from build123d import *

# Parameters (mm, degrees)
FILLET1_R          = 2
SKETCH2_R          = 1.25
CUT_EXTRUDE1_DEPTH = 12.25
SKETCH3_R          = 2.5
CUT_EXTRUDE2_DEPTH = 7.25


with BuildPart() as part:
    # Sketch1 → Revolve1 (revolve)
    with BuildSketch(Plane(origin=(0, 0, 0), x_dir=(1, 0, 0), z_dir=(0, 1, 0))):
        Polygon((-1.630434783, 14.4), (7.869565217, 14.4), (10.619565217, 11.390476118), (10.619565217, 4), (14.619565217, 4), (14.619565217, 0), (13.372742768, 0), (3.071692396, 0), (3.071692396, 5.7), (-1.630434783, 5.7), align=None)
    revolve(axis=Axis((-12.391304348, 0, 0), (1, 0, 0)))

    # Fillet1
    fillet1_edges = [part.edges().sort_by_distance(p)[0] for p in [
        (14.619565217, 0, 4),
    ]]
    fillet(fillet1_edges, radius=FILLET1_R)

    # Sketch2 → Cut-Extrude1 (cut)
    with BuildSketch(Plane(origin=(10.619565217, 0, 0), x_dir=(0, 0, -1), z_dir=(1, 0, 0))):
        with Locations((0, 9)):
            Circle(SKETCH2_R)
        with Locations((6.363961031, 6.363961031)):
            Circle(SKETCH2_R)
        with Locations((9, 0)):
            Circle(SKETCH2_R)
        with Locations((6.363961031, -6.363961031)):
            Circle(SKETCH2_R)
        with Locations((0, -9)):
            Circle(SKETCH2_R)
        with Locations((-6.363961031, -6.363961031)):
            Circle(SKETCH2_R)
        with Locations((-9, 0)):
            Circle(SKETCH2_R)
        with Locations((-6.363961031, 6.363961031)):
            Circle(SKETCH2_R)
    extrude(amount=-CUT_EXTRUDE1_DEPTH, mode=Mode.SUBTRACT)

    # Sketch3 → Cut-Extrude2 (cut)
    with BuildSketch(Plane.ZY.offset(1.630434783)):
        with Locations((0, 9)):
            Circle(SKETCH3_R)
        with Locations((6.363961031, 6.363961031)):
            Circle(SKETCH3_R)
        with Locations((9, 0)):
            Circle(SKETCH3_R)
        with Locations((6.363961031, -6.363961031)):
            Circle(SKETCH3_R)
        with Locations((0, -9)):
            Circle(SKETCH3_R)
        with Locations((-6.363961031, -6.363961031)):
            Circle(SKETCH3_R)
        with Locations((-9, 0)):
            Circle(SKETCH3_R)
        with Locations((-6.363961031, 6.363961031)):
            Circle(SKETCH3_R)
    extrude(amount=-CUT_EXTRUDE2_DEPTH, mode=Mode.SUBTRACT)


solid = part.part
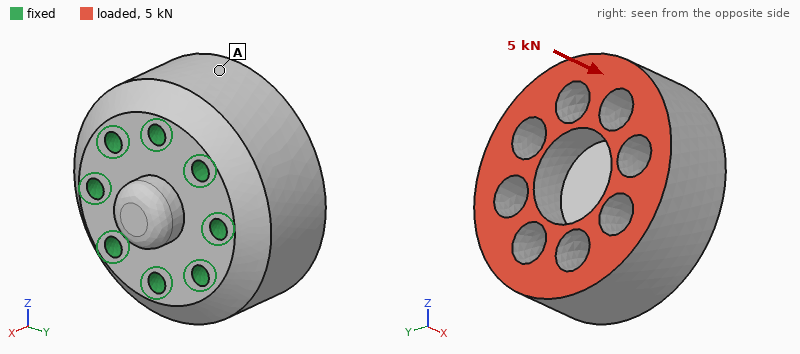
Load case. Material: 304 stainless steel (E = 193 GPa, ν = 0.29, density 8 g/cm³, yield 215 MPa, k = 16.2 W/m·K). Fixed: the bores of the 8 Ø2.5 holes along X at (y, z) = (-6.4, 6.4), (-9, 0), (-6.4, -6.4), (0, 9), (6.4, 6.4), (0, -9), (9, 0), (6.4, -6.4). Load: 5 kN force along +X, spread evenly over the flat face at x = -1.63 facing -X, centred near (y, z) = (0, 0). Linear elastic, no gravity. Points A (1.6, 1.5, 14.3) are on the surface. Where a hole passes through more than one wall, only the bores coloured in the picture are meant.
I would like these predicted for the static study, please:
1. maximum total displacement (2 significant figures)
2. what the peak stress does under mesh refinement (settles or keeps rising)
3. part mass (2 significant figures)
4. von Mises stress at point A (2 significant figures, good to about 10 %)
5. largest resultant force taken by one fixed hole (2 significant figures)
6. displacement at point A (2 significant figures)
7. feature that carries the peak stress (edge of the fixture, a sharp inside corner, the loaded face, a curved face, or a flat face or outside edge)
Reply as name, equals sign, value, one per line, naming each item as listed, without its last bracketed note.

maximum total displacement = 1.4 µm
what the peak stress does under mesh refinement = keeps rising
part mass = 48 g
von Mises stress at point A = 13 MPa
largest resultant force taken by one fixed hole = 630 N
displacement at point A = 1.1 µm
feature that carries the peak stress = edge of the fixture
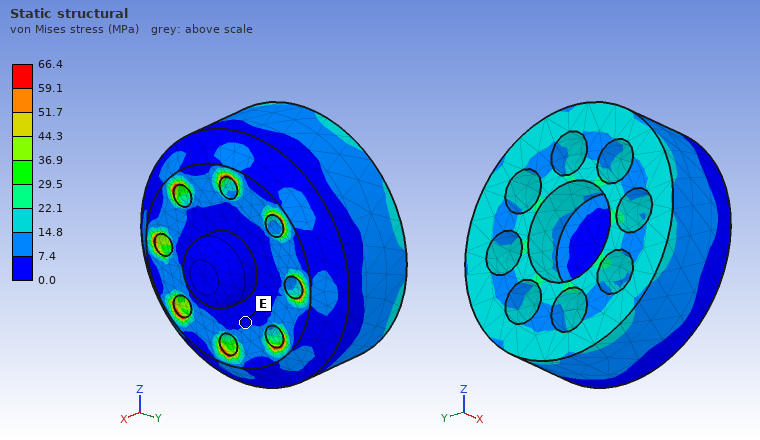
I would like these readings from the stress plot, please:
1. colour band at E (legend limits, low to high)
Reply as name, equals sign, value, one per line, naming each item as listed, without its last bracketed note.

colour band at E = 0.0 to 7.4 MPa
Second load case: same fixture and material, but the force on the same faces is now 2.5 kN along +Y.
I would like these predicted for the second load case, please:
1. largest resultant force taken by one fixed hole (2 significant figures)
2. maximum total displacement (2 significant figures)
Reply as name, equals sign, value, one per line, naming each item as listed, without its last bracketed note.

largest resultant force taken by one fixed hole = 530 N
maximum total displacement = 3.1 µm
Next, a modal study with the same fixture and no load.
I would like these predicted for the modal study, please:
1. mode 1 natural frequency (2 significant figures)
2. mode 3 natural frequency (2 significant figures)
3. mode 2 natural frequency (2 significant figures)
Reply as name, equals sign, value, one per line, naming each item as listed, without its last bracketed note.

mode 1 natural frequency = 47 kHz
mode 3 natural frequency = 51 kHz
mode 2 natural frequency = 47 kHz
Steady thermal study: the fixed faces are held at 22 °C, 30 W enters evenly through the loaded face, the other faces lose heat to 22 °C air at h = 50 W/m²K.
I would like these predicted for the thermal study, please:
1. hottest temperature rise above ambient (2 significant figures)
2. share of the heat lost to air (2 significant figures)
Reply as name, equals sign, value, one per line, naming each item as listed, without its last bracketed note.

hottest temperature rise above ambient = 46 K
share of the heat lost to air = 9.7 %
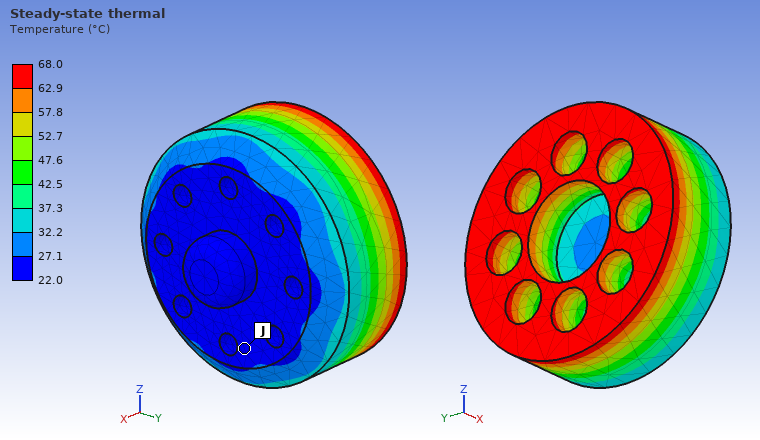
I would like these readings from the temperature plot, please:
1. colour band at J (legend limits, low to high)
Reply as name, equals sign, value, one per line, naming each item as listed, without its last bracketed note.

colour band at J = 22.0 to 27.1 °C
